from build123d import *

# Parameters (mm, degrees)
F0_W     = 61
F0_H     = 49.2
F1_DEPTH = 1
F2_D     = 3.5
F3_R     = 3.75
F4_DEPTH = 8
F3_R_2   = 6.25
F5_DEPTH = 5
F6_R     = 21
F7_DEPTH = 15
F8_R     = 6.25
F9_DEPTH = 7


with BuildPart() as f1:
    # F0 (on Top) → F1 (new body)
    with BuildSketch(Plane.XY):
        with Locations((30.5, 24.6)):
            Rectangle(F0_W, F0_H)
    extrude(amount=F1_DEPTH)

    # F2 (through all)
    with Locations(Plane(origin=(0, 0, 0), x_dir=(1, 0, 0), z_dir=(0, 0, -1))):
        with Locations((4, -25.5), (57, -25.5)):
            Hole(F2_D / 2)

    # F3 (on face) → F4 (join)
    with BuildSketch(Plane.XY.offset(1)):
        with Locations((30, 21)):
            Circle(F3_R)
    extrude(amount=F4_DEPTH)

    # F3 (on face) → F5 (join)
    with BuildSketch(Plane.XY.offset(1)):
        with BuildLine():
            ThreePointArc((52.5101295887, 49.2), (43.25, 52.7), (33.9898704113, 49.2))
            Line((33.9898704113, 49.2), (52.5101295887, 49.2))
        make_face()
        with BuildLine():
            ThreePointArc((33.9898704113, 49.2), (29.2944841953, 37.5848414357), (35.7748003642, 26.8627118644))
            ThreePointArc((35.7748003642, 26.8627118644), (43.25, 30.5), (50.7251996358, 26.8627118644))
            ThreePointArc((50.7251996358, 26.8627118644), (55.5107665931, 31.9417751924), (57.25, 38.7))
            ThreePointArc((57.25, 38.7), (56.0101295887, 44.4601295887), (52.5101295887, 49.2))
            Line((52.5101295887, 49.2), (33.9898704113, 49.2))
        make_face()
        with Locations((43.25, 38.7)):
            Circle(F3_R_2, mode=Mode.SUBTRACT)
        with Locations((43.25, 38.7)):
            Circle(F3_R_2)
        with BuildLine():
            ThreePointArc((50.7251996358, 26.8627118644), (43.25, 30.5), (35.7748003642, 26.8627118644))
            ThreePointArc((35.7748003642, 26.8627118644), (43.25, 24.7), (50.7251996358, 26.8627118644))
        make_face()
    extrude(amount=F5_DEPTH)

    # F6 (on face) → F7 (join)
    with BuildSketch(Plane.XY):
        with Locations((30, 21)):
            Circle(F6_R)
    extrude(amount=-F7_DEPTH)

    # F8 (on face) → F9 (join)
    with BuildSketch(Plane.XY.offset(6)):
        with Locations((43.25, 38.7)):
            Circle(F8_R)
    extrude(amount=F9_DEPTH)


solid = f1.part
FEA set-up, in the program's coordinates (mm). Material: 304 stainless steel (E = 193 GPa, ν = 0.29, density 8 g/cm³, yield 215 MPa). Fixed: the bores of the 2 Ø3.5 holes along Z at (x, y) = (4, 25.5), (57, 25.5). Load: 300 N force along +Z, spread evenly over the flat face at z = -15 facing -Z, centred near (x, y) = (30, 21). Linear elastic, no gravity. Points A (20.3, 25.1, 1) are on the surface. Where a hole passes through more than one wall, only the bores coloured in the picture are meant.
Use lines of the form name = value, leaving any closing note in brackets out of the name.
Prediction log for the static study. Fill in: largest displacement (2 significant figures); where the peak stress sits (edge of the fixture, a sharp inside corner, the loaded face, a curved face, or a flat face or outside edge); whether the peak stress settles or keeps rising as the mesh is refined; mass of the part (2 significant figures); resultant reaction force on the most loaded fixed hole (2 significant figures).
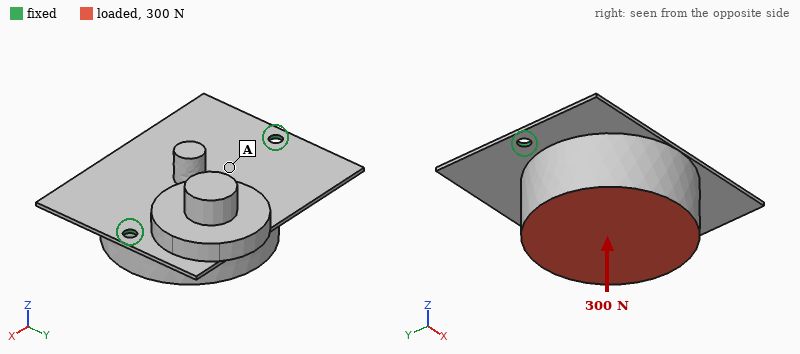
largest displacement = 0.12 mm
where the peak stress sits = edge of the fixture
whether the peak stress settles or keeps rising as the mesh is refined = keeps rising
mass of the part = 220 g
resultant reaction force on the most loaded fixed hole = 170 N
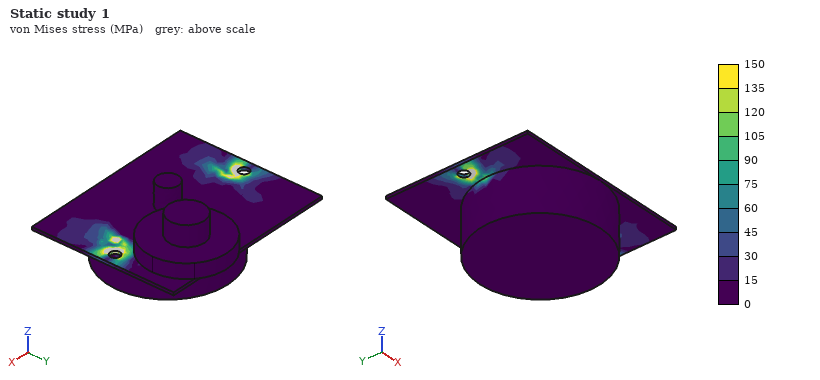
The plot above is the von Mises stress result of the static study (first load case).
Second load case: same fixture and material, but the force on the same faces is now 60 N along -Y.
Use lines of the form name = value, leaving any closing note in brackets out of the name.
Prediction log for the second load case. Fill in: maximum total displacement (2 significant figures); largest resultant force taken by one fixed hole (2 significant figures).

maximum total displacement = 75 µm
largest resultant force taken by one fixed hole = 35 N
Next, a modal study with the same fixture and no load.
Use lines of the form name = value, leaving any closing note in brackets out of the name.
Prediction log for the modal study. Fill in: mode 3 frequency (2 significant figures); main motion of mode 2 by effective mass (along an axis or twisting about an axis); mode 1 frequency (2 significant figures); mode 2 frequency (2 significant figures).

mode 3 frequency = 3400 Hz
main motion of mode 2 by effective mass = along Z
mode 1 frequency = 450 Hz
mode 2 frequency = 2100 Hz
